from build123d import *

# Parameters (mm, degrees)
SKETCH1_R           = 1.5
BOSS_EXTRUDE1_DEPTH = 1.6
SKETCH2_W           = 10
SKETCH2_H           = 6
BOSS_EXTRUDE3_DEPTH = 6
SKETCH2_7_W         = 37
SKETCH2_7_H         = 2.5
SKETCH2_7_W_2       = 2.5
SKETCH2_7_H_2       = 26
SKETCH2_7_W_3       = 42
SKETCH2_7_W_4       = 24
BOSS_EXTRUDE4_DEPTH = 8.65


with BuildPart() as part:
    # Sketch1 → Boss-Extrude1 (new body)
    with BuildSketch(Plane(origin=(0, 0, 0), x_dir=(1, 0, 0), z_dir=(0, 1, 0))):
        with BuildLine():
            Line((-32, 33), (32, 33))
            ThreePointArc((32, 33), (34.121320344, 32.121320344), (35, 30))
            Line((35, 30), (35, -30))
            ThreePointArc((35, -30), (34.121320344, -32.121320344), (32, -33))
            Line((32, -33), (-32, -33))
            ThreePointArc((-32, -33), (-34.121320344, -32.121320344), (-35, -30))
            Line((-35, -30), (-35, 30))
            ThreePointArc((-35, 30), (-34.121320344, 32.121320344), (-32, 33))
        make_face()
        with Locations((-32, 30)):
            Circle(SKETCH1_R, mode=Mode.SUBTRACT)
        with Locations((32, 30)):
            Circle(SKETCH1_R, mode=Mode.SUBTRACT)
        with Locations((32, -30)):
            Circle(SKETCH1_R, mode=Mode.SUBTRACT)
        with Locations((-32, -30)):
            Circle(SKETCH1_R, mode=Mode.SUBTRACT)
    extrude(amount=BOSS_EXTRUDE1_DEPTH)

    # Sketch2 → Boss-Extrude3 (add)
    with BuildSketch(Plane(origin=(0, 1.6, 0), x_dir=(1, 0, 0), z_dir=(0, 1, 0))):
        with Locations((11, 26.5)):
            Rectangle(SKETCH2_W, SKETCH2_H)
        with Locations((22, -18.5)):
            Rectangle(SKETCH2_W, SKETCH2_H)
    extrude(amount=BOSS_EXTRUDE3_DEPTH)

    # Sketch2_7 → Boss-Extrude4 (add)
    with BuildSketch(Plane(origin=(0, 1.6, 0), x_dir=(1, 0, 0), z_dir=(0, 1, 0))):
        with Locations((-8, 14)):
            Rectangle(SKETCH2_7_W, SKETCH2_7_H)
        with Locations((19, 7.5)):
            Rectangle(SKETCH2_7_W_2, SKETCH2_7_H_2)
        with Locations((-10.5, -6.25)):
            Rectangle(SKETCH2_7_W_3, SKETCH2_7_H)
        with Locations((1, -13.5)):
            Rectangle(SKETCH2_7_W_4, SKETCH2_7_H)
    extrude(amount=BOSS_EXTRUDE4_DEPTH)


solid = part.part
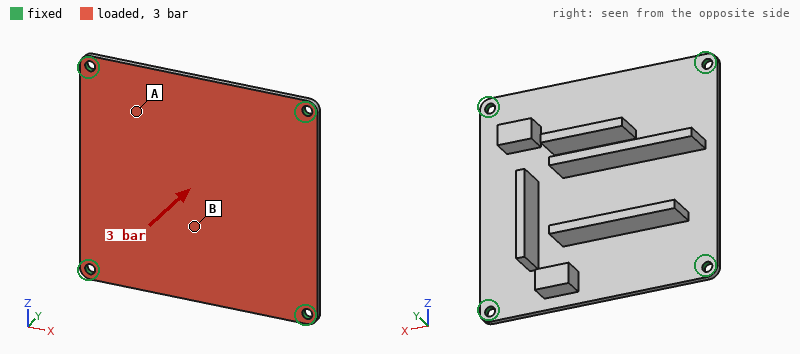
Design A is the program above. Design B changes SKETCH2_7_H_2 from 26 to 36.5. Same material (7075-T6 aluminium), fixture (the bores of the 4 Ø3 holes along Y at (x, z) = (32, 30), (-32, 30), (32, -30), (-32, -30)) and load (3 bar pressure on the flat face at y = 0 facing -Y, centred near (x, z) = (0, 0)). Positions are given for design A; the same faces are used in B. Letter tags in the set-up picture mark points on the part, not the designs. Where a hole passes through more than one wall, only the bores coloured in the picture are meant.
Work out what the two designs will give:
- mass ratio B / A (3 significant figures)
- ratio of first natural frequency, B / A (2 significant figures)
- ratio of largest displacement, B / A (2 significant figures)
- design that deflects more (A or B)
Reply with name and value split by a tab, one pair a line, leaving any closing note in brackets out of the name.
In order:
mass ratio B / A	1.02
ratio of first natural frequency, B / A	1.0
ratio of largest displacement, B / A	0.86
design that deflects more	A
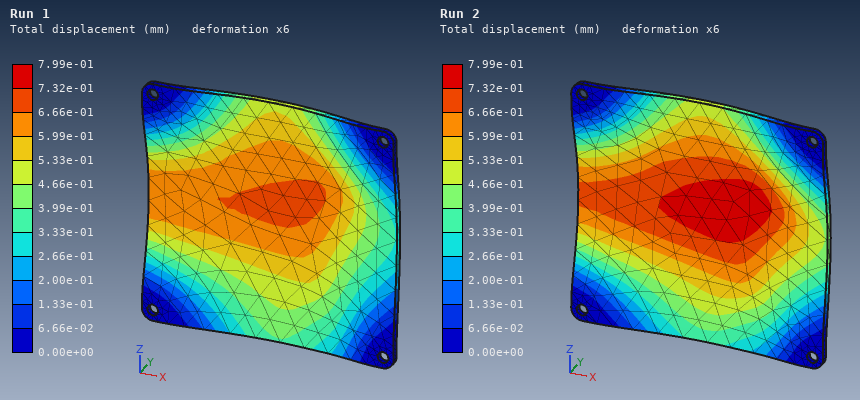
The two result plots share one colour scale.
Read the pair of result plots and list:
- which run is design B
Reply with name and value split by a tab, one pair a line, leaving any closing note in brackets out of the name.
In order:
which run is design B	Run 1
